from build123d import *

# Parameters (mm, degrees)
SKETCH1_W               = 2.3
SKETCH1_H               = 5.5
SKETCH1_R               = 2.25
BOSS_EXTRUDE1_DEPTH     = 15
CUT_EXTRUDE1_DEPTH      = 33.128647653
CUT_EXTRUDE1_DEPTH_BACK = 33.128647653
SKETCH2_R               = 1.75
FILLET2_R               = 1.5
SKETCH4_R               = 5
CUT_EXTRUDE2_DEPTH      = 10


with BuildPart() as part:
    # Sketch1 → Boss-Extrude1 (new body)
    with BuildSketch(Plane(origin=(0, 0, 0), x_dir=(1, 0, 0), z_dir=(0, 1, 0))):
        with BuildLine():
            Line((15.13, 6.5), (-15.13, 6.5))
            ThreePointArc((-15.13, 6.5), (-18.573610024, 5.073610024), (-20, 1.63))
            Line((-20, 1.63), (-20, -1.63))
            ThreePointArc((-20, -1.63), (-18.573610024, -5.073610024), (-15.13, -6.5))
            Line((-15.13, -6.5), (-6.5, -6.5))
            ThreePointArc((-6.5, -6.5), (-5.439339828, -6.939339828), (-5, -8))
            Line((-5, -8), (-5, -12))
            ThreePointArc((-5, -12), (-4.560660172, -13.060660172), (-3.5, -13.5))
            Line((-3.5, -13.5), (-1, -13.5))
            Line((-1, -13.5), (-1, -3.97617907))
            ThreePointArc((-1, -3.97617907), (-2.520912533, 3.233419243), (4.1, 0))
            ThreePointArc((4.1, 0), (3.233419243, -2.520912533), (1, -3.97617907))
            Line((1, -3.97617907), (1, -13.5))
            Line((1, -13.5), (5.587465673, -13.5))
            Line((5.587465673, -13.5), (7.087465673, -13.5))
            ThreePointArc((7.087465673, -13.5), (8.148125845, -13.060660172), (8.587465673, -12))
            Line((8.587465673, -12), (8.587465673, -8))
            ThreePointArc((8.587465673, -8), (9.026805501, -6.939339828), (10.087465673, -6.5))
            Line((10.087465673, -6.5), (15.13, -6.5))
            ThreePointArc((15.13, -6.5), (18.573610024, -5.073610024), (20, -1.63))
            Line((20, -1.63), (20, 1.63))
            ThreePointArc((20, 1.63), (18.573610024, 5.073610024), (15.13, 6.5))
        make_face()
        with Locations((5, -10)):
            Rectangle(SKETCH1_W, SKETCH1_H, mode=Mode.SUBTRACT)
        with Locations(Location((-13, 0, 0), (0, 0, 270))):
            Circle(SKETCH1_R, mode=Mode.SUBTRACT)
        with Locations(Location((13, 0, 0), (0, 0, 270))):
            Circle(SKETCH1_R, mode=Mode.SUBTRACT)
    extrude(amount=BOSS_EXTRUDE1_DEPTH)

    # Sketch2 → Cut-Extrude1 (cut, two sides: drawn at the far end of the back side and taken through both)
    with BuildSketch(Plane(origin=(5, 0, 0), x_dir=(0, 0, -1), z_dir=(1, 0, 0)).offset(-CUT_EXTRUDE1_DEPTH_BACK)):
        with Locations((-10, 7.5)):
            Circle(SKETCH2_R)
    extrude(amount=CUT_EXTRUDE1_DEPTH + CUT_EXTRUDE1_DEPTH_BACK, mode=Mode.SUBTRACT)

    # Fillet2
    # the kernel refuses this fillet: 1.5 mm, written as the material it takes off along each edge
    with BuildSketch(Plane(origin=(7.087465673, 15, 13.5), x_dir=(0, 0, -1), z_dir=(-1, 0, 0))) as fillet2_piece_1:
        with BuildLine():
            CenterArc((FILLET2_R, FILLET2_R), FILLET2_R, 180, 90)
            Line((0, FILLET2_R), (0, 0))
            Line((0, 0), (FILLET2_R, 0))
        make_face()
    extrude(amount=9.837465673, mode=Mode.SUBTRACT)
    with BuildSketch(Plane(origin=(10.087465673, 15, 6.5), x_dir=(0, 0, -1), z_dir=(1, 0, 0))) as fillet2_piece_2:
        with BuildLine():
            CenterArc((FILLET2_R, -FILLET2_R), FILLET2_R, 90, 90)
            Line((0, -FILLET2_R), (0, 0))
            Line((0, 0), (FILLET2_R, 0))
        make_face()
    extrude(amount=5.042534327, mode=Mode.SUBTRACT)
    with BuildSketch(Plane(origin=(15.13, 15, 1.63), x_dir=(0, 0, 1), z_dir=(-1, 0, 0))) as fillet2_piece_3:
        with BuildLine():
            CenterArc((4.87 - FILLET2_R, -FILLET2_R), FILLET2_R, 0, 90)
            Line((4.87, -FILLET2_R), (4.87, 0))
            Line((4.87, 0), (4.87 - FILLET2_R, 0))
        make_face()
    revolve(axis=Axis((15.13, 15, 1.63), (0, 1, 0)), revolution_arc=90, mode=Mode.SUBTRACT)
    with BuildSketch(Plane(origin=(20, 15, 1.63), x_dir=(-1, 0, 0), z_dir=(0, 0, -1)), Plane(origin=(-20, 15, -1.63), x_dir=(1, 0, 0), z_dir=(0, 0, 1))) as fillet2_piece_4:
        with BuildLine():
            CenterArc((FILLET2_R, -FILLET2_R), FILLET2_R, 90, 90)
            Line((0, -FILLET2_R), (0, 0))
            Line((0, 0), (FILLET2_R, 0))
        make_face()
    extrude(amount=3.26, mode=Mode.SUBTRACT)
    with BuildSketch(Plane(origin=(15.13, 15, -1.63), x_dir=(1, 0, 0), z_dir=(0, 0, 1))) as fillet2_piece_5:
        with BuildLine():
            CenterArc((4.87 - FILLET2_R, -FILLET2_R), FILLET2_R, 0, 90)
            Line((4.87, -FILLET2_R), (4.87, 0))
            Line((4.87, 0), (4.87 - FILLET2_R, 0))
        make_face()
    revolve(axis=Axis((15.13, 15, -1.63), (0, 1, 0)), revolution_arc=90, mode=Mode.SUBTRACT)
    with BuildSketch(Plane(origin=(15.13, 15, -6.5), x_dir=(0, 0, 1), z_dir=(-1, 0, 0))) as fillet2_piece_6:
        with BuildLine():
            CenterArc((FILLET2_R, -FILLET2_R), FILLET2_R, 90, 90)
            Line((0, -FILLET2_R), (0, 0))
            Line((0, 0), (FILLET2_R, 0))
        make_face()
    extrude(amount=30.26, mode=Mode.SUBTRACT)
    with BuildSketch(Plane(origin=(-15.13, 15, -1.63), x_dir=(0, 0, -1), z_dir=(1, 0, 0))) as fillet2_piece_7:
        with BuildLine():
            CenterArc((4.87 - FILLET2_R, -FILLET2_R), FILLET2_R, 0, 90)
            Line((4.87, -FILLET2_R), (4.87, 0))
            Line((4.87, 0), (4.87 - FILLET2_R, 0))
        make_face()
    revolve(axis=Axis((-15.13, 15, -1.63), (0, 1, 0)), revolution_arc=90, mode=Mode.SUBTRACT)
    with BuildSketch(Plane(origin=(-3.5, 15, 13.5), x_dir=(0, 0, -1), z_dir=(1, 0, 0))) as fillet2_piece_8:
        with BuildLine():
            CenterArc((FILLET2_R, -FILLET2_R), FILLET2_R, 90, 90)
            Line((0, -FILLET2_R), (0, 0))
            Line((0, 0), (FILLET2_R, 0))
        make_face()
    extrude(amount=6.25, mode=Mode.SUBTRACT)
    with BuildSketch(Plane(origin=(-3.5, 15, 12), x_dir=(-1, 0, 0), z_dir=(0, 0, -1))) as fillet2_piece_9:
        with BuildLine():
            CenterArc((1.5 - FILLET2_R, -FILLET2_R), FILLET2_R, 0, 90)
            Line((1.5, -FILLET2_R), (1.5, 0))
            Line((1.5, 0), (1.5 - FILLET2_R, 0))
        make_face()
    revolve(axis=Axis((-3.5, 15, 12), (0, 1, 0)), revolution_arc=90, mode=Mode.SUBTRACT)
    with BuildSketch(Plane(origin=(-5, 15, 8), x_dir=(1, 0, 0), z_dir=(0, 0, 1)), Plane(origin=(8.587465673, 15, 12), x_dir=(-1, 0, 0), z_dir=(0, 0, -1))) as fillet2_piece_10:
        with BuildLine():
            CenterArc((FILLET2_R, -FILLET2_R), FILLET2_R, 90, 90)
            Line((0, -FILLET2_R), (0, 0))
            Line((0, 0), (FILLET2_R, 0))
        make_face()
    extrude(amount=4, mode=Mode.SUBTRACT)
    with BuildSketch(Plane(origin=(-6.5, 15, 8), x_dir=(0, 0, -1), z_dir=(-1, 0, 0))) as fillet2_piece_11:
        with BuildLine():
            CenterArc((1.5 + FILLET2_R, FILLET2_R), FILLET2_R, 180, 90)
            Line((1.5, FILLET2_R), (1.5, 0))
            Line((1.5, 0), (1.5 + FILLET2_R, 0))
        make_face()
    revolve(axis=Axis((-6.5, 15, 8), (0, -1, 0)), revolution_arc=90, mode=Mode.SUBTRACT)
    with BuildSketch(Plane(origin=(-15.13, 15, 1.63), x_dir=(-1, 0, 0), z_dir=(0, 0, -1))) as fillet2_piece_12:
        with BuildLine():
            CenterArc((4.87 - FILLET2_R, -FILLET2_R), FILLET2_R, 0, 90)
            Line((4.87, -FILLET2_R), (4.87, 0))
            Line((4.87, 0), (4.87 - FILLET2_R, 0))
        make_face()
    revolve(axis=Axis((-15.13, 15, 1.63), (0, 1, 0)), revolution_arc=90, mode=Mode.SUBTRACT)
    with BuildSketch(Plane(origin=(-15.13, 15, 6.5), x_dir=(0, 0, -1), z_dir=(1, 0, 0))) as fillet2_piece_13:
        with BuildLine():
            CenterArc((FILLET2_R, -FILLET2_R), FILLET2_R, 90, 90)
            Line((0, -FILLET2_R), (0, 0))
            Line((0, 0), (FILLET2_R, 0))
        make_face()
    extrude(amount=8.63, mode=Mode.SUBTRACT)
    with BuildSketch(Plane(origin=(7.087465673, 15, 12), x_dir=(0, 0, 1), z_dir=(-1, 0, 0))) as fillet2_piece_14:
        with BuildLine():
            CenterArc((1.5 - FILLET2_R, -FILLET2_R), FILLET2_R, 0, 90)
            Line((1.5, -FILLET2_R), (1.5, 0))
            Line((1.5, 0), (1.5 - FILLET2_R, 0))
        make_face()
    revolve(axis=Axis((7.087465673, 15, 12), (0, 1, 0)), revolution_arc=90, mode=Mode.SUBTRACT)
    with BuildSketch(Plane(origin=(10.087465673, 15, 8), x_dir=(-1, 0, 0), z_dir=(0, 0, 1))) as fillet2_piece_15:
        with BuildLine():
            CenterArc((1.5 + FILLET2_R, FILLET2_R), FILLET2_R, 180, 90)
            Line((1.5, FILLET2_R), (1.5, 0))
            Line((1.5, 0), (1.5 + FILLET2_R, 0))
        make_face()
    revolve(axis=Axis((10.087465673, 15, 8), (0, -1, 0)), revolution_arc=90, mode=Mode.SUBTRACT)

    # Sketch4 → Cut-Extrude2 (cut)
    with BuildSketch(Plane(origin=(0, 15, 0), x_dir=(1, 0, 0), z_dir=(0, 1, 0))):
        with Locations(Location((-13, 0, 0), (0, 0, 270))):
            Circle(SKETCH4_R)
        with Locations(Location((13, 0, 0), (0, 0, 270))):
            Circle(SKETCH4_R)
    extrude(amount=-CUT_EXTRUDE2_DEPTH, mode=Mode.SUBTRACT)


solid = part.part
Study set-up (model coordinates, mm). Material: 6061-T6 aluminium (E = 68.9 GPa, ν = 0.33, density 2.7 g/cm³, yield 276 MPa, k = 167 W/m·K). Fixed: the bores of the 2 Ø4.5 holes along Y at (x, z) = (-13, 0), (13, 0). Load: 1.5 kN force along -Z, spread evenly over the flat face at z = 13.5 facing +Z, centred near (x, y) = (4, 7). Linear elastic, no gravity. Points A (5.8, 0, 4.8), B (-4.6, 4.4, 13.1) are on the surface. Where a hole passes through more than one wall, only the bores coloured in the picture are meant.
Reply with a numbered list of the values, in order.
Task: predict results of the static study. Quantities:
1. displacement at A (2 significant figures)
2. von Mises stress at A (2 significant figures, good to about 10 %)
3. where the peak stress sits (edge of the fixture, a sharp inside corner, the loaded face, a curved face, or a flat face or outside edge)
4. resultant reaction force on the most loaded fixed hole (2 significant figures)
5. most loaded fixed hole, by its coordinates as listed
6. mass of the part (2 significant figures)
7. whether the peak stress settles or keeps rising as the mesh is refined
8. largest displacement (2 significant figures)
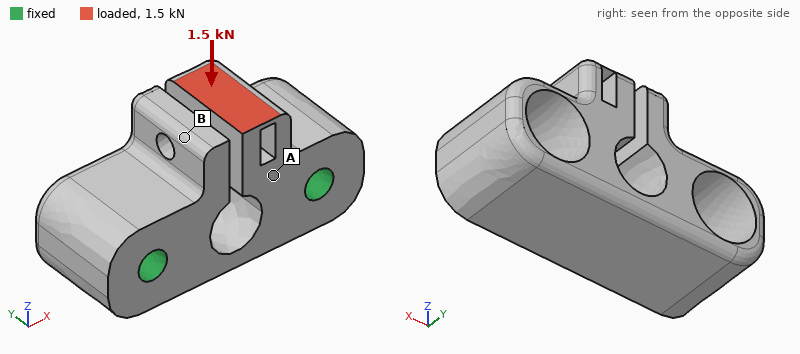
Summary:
1. 10 µm
2. 21 MPa
3. edge of the fixture
4. 1.3 kN
5. (13, 0)
6. 16 g
7. keeps rising
8. 40 µm
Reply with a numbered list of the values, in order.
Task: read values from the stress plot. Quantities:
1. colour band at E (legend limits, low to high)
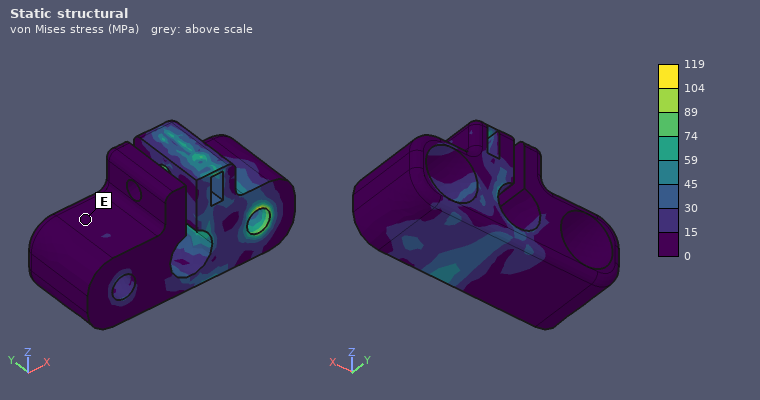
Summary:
1. 0 to 15 MPa
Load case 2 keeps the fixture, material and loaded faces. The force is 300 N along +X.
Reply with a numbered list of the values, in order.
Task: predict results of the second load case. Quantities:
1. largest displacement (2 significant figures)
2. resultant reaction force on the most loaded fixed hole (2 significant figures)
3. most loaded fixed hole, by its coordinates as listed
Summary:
1. 24 µm
2. 410 N
3. (13, 0)
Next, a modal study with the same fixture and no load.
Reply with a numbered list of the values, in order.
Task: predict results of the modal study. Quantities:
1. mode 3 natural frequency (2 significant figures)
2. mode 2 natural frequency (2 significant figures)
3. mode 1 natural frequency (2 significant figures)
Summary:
1. 17 kHz
2. 16 kHz
3. 14 kHz
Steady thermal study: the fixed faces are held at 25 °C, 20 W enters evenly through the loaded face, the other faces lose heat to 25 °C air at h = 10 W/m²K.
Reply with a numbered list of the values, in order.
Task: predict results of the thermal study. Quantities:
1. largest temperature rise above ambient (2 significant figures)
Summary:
1. 29 K
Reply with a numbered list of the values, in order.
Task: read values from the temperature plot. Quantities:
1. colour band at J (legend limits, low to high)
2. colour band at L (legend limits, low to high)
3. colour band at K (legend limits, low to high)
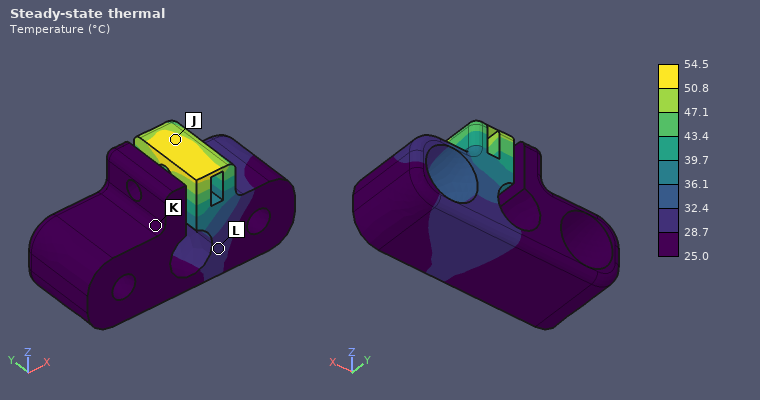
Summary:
1. 50.8 to 54.5 °C
2. 28.7 to 32.4 °C
3. 25.0 to 28.7 °C
